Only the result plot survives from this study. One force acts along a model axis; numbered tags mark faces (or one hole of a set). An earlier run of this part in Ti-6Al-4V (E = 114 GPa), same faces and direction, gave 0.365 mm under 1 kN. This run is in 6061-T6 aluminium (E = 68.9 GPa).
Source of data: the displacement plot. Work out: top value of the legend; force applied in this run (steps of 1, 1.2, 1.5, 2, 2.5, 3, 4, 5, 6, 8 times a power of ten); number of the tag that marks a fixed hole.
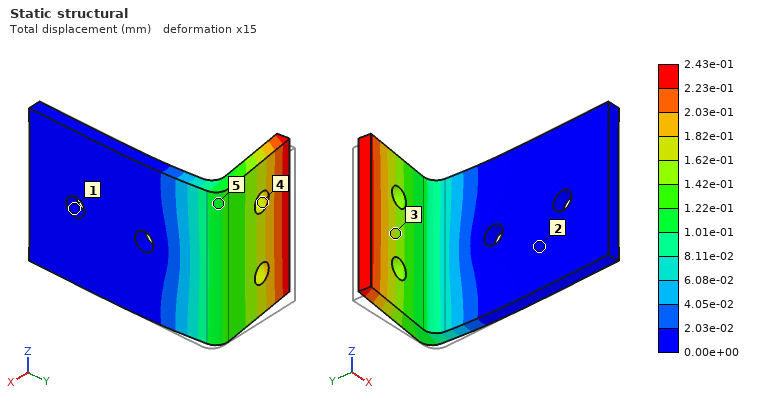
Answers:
2.43e-01 mm
400 N
1
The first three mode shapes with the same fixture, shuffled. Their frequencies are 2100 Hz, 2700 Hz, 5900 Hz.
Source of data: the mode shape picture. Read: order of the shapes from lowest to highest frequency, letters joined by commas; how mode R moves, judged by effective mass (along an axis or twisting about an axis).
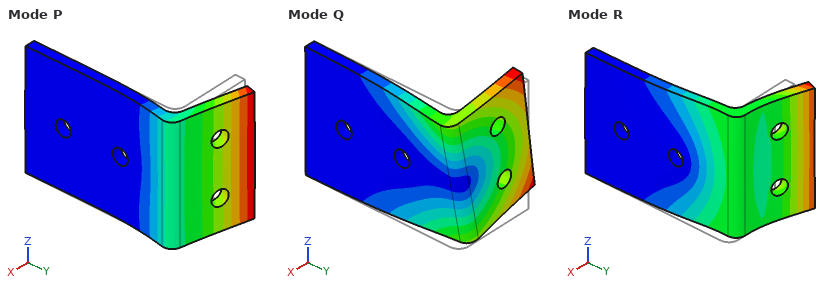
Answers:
P, Q, R
along X
